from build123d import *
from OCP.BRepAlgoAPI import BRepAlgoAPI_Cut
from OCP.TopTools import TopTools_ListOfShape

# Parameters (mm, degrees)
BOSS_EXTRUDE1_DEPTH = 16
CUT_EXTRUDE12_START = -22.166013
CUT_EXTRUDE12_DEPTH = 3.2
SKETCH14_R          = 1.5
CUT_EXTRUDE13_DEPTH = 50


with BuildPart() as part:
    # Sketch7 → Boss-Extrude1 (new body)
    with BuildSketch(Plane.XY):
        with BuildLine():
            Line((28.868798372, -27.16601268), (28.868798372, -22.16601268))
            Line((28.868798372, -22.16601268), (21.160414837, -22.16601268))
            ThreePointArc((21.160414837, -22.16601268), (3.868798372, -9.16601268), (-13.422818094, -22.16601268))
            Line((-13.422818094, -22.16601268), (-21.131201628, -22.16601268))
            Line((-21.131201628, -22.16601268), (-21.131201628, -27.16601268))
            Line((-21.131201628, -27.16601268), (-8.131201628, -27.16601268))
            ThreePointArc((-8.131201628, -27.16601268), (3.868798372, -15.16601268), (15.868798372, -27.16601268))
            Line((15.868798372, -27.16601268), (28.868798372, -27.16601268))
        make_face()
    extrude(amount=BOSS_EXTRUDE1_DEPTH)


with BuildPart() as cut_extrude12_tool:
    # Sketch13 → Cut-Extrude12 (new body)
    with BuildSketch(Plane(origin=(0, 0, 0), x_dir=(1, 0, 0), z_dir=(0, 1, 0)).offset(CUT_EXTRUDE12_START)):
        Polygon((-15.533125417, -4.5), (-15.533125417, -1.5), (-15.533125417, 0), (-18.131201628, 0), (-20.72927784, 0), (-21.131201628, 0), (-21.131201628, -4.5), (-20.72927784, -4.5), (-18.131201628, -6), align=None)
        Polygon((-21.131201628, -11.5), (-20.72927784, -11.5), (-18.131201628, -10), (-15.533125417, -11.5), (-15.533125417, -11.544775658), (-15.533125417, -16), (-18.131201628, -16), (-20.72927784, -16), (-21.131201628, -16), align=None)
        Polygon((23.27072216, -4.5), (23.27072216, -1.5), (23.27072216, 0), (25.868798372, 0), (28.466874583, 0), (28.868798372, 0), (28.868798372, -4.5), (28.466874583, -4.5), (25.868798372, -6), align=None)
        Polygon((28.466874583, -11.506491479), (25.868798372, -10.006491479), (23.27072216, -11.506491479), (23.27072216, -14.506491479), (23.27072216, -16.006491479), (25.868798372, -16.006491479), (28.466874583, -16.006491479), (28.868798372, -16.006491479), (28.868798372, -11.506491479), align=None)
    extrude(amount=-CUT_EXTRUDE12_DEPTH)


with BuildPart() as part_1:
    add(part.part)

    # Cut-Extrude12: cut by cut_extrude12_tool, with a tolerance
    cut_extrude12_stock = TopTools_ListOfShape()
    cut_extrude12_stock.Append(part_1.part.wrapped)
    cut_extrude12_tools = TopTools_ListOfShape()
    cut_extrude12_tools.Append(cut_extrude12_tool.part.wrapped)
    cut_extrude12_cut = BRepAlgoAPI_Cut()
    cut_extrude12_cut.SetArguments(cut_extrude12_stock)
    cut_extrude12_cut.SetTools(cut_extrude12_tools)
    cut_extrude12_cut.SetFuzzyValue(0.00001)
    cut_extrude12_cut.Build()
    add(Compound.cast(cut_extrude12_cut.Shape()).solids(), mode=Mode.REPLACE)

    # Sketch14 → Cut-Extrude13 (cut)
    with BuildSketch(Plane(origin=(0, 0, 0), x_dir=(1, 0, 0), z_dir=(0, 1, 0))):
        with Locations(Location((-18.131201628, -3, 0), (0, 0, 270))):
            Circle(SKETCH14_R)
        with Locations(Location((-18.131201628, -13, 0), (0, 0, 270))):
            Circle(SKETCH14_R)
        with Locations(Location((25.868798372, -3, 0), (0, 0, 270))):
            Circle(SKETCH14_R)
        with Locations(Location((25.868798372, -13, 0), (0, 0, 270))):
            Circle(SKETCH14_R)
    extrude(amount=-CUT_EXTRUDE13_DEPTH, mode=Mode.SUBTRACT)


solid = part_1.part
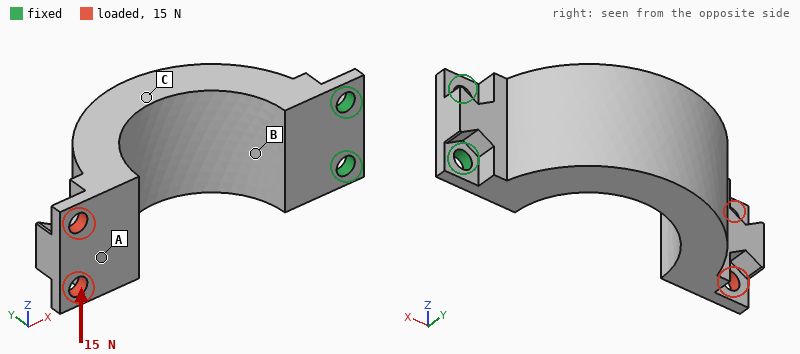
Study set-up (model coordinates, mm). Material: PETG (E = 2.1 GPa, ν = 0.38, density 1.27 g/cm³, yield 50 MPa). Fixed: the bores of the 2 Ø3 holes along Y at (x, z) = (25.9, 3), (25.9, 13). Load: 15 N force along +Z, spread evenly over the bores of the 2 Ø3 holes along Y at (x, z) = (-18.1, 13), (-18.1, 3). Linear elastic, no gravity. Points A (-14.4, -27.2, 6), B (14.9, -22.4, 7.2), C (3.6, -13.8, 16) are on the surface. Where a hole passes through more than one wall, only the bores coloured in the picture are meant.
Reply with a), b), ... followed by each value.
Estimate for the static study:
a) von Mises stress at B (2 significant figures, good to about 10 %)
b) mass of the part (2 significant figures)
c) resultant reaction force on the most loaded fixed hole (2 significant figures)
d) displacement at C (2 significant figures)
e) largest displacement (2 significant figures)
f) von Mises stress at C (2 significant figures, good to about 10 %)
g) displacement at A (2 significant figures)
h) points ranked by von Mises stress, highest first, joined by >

a) 5.9 MPa
b) 6.7 g
c) 58 N
d) 0.17 mm
e) 0.61 mm
f) 2.4 MPa
g) 0.50 mm
h) B > C > A
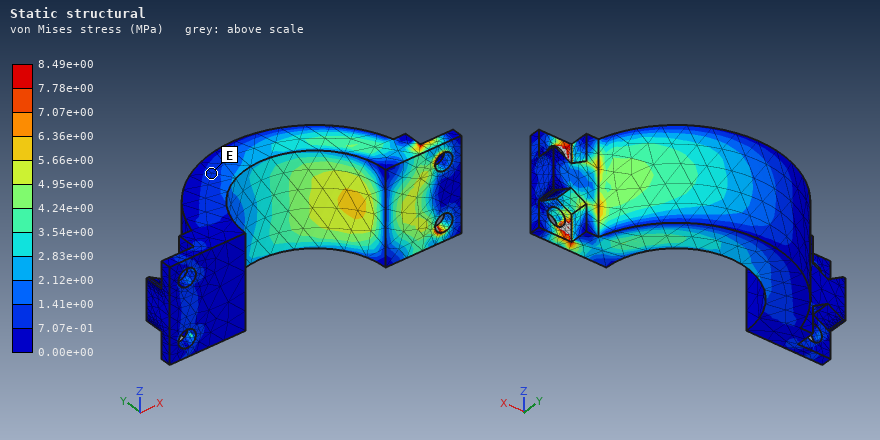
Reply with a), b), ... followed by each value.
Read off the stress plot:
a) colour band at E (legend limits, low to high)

a) 7.07e-01 to 1.41e+00 MPa
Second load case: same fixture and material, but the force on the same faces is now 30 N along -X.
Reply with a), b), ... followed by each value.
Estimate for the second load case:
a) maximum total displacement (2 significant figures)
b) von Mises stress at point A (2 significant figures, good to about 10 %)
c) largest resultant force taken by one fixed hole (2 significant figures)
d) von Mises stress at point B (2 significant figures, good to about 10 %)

a) 0.58 mm
b) 0.92 MPa
c) 15 N
d) 2.0 MPa
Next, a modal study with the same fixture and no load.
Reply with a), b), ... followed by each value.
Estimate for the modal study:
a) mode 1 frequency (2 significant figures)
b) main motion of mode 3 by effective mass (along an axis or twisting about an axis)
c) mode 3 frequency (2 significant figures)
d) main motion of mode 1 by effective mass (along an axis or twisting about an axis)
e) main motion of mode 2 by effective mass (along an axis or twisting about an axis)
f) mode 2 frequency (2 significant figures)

a) 270 Hz
b) along X
c) 1300 Hz
d) along Y
e) along Z
f) 700 Hz
